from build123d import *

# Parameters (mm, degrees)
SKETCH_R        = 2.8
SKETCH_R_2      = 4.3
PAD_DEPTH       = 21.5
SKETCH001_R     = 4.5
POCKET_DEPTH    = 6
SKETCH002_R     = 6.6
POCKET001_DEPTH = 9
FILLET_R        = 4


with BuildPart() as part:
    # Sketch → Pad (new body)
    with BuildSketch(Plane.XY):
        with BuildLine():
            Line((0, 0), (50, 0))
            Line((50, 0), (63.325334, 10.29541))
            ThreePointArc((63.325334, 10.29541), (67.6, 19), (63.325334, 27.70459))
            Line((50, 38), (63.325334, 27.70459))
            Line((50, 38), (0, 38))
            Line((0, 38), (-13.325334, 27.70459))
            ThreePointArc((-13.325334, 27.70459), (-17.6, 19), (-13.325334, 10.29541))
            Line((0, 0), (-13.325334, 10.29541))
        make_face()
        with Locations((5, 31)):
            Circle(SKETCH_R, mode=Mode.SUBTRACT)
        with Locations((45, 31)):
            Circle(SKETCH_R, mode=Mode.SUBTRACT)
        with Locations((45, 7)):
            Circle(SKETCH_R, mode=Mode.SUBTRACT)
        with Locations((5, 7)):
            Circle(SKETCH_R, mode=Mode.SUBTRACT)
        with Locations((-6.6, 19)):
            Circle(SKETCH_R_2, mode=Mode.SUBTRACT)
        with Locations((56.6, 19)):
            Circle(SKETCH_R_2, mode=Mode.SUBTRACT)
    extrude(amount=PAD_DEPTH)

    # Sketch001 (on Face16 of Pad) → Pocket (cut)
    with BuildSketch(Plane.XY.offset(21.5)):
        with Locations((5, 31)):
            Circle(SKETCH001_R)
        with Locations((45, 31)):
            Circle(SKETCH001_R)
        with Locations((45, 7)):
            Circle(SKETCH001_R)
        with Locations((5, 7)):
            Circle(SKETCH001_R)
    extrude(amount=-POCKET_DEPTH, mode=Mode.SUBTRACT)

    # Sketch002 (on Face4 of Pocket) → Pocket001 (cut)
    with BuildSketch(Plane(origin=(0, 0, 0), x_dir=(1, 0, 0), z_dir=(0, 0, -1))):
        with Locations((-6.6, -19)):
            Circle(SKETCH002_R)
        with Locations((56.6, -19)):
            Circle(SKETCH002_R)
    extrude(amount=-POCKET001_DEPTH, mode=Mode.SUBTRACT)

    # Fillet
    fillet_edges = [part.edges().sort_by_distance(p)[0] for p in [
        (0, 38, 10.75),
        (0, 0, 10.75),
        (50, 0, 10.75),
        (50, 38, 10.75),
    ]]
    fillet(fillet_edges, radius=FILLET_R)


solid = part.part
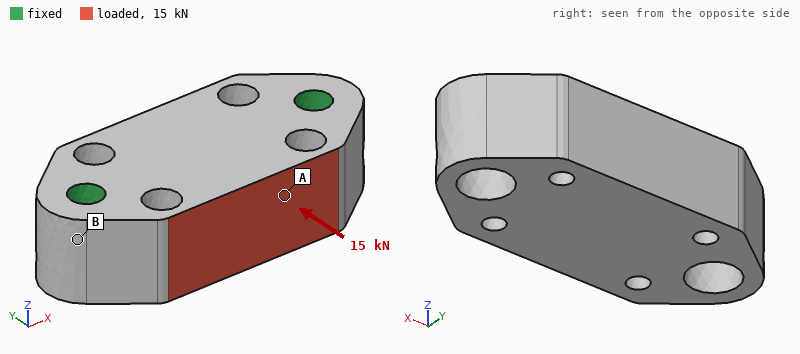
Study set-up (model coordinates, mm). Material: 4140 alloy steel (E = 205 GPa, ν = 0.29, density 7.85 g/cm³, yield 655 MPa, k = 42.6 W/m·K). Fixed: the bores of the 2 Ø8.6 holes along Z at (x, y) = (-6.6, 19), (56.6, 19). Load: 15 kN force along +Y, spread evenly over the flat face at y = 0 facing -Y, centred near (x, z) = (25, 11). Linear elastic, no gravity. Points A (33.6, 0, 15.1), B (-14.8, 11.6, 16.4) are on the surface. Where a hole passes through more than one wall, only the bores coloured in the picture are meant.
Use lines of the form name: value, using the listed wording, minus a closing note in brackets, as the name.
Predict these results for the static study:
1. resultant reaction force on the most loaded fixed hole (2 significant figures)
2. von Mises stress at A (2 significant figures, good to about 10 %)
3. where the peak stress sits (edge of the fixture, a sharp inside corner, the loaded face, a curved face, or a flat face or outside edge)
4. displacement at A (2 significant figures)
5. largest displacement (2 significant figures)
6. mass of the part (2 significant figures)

resultant reaction force on the most loaded fixed hole: 7.6 kN
von Mises stress at A: 21 MPa
where the peak stress sits: edge of the fixture
displacement at A: 6.8 µm
largest displacement: 9.6 µm
mass of the part: 410 g
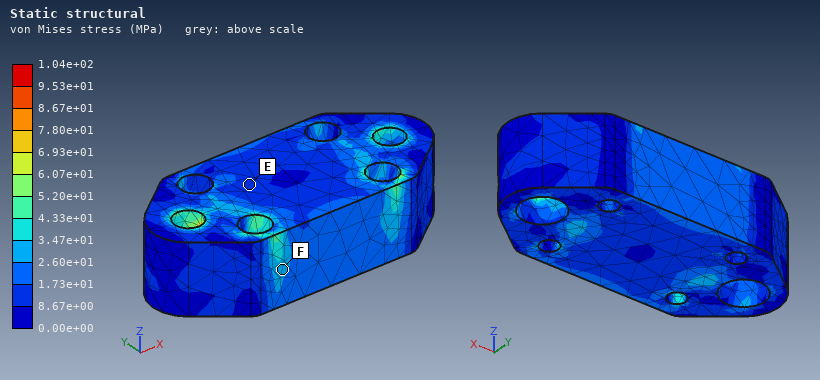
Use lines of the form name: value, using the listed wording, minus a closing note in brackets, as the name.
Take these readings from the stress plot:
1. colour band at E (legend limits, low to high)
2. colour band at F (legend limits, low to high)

colour band at E: 8.67e+00 to 1.73e+01 MPa
colour band at F: 2.60e+01 to 3.47e+01 MPa
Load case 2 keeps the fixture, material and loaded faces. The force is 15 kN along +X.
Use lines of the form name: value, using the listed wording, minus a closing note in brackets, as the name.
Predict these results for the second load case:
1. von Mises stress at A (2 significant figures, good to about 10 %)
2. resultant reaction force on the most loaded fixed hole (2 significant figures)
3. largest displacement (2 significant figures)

von Mises stress at A: 26 MPa
resultant reaction force on the most loaded fixed hole: 8.7 kN
largest displacement: 5.5 µm
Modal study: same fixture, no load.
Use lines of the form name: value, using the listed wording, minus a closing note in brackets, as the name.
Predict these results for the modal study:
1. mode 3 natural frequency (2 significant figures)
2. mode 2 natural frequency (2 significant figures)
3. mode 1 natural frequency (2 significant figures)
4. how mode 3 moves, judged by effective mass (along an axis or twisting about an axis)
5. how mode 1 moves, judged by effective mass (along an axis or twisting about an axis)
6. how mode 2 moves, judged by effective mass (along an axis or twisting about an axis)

mode 3 natural frequency: 16 kHz
mode 2 natural frequency: 13 kHz
mode 1 natural frequency: 11 kHz
how mode 3 moves, judged by effective mass: along Y
how mode 1 moves, judged by effective mass: along Y
how mode 2 moves, judged by effective mass: along Z
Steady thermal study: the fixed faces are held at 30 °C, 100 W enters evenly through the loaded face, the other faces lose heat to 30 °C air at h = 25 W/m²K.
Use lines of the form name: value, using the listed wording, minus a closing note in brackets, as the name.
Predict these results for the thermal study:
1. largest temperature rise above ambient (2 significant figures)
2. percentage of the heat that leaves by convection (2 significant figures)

largest temperature rise above ambient: 72 K
percentage of the heat that leaves by convection: 7.0 %
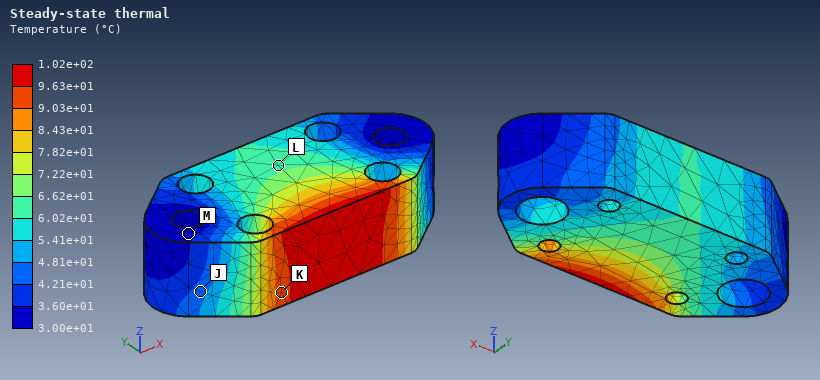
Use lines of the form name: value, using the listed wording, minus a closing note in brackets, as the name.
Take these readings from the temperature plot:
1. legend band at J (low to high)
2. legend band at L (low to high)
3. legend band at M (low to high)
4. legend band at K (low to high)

legend band at J: 4.21e+01 to 4.81e+01 °C
legend band at L: 6.02e+01 to 6.62e+01 °C
legend band at M: 3.00e+01 to 3.60e+01 °C
legend band at K: 9.03e+01 to 9.63e+01 °C
